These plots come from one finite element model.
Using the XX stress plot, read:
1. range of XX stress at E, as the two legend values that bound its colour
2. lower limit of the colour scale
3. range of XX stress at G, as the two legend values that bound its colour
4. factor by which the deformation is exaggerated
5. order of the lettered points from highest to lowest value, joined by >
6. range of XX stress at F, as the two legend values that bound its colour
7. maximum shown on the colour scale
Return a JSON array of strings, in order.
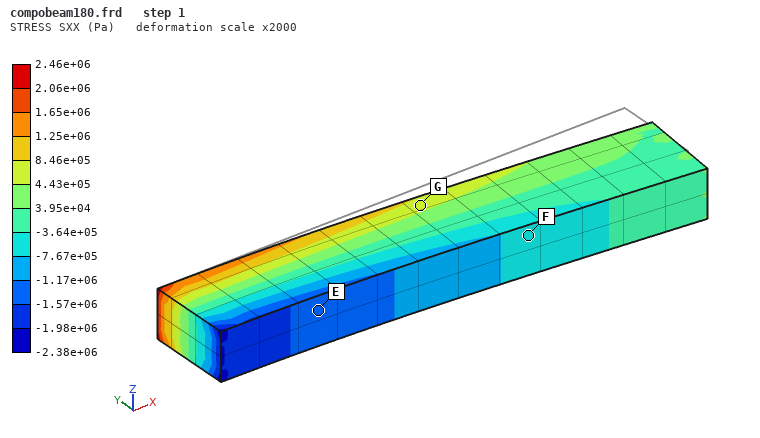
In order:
["-1.57e+06 to -1.17e+06 Pa", "-2.38e+06 Pa", "4.43e+05 to 8.46e+05 Pa", "2000", "G > F > E", "-7.67e+05 to -3.64e+05 Pa", "2.46e+06 Pa"]
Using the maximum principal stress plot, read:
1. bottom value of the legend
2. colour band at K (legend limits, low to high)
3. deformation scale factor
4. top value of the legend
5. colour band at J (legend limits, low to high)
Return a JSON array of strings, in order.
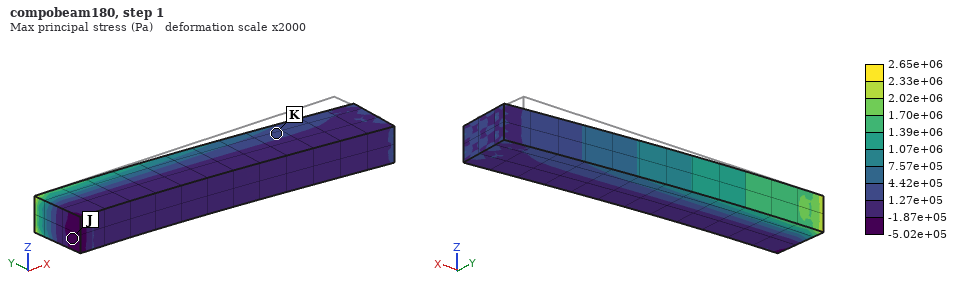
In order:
["-5.02e+05 Pa", "1.27e+05 to 4.42e+05 Pa", "2000", "2.65e+06 Pa", "-5.02e+05 to -1.87e+05 Pa"]
